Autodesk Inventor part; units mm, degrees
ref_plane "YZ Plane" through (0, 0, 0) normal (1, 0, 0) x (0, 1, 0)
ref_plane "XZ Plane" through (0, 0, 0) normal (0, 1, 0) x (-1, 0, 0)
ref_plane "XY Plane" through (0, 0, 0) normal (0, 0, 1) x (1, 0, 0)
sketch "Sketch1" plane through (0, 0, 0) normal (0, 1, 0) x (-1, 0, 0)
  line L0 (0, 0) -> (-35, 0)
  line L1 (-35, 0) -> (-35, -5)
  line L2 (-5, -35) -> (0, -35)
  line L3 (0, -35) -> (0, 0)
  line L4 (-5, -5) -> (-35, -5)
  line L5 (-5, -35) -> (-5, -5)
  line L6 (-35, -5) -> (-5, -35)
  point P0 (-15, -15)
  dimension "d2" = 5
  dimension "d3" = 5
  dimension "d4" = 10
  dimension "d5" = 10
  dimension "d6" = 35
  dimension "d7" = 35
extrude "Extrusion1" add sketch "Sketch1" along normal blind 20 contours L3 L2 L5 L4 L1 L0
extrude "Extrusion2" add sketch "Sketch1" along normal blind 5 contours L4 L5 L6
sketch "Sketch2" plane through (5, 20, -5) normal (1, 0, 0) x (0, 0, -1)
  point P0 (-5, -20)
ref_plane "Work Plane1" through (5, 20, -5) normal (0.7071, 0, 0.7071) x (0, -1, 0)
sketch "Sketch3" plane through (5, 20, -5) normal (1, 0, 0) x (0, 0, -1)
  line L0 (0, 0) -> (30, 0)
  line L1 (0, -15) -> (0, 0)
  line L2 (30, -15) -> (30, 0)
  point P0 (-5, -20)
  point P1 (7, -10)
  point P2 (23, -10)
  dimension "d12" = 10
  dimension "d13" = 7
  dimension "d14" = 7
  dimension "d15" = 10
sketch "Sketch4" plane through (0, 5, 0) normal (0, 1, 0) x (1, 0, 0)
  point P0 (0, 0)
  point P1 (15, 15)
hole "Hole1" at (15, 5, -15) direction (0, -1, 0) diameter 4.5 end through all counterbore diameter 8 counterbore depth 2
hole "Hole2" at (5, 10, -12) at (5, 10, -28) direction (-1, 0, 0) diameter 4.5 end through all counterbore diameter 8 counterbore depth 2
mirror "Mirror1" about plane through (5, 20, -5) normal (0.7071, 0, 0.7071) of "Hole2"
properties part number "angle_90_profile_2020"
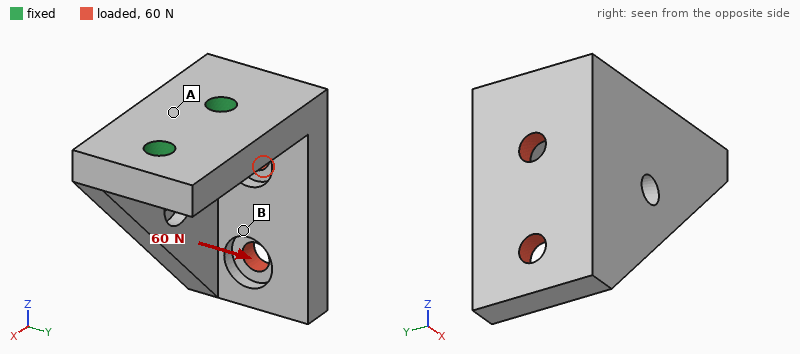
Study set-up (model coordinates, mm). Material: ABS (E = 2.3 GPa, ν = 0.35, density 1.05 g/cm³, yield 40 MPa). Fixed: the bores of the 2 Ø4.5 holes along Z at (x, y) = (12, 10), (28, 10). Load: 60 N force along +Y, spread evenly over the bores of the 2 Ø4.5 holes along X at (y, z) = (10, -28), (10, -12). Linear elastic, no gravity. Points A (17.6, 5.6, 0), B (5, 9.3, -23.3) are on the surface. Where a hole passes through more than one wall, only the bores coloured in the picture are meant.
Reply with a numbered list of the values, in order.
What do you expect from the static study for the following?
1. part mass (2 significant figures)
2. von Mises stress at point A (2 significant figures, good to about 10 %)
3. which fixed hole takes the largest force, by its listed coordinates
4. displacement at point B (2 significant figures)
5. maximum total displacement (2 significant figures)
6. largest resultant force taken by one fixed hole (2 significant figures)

1. 8.4 g
2. 5.4 MPa
3. (12, 10)
4. 0.34 mm
5. 0.54 mm
6. 81 N
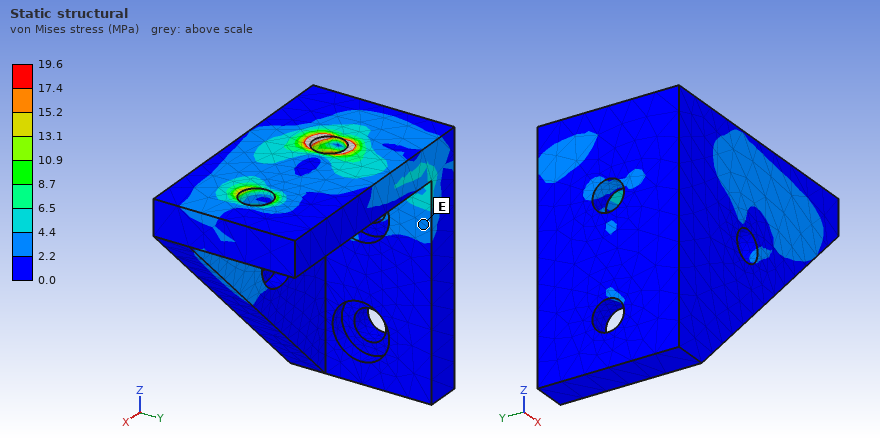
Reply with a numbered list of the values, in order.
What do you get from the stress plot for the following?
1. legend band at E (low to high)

1. 2.2 to 4.4 MPa
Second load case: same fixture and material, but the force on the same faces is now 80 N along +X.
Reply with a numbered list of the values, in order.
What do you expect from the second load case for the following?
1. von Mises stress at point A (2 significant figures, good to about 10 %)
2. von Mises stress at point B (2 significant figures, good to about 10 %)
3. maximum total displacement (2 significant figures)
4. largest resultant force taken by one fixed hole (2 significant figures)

1. 2.4 MPa
2. 3.0 MPa
3. 0.37 mm
4. 91 N
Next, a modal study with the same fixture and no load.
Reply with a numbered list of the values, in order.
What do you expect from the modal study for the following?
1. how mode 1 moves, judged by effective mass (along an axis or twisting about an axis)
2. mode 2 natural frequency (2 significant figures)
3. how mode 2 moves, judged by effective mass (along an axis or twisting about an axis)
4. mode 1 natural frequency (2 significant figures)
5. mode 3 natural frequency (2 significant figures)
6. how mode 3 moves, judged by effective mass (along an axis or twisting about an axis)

1. along Y
2. 1700 Hz
3. along X
4. 990 Hz
5. 3400 Hz
6. along Z
